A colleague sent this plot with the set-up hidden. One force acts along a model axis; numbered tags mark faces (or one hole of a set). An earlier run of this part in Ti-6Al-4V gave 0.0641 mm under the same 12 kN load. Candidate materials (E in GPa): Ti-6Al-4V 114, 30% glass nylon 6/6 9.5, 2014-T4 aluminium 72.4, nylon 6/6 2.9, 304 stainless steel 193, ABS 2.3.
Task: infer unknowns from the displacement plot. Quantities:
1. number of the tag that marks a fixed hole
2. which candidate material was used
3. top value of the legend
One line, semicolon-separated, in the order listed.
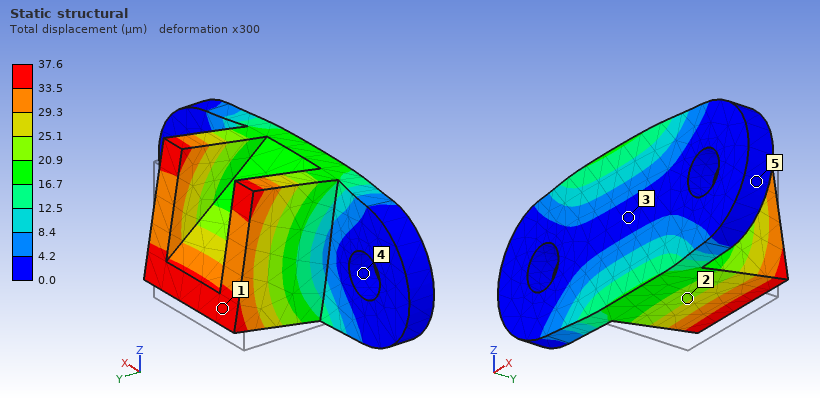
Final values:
4; 304 stainless steel; 37.6 µm
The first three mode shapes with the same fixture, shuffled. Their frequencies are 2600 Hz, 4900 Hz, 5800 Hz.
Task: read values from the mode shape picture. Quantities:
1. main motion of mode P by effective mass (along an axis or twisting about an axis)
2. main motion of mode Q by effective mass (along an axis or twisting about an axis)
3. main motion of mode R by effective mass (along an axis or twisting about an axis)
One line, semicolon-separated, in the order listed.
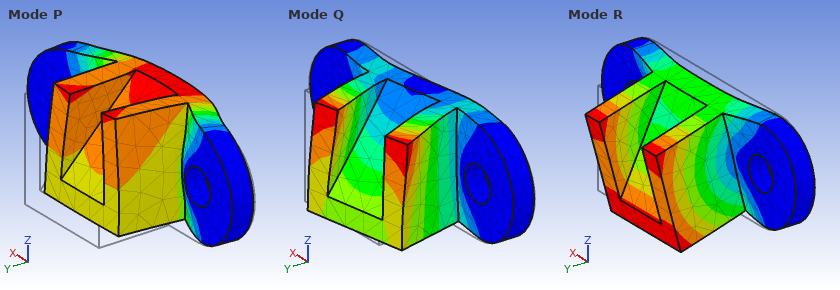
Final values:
along Y; along X; along Z
